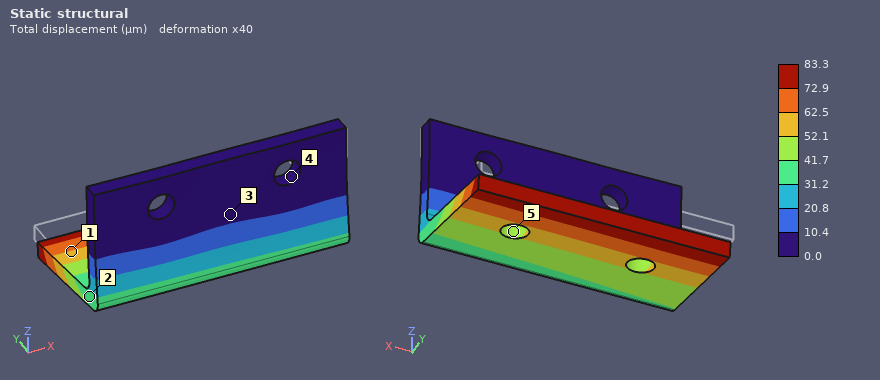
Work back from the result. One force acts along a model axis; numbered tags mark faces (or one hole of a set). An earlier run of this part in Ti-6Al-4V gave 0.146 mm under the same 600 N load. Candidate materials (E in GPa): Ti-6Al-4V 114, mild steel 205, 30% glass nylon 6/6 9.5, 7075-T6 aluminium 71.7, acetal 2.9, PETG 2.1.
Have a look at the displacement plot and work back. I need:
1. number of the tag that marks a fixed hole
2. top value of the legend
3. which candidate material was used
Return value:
4
83.3 µm
mild steel
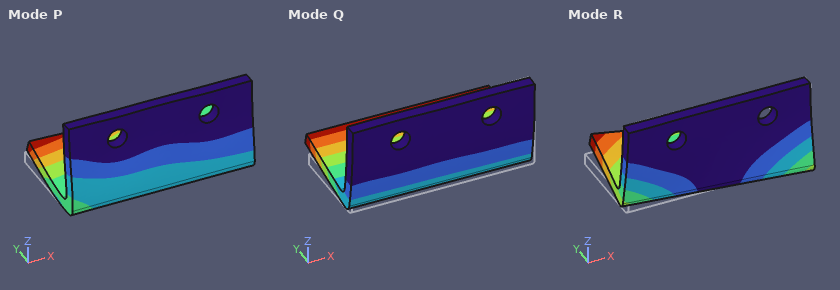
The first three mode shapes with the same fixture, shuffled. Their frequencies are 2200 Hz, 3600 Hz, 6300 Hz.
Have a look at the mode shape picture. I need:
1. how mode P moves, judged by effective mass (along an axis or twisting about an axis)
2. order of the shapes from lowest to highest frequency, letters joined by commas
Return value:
along Y
Q, R, P
